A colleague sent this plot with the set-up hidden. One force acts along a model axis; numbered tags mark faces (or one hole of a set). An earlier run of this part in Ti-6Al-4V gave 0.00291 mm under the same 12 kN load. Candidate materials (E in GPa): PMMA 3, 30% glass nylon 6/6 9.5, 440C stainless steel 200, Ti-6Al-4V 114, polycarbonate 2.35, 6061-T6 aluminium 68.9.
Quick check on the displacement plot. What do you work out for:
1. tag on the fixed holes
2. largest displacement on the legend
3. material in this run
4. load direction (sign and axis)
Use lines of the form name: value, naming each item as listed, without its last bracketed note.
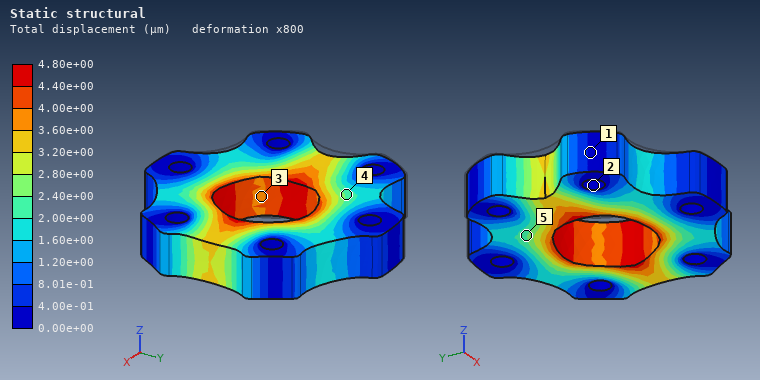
tag on the fixed holes: 2
largest displacement on the legend: 4.80e+00 µm
material in this run: 6061-T6 aluminium
load direction: +X
